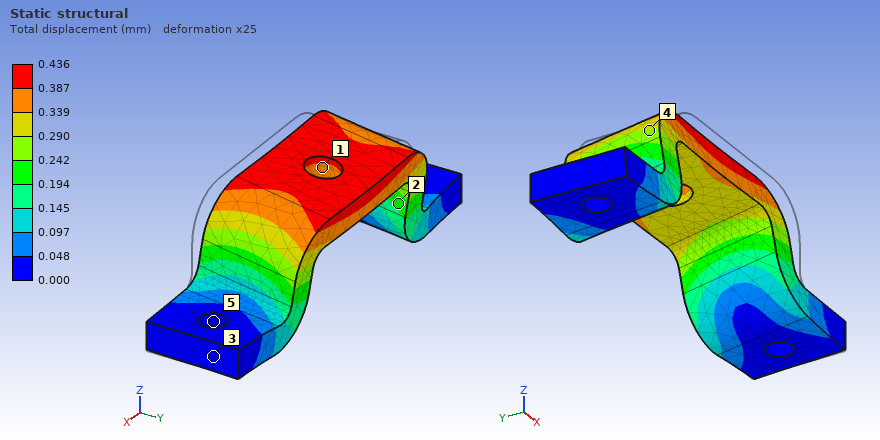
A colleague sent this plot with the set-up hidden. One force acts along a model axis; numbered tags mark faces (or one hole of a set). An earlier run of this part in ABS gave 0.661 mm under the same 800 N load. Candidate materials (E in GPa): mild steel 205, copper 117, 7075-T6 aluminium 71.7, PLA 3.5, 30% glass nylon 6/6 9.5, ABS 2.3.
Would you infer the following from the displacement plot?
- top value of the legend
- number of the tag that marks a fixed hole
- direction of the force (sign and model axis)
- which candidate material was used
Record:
0.436 mm
5
+Y
PLA
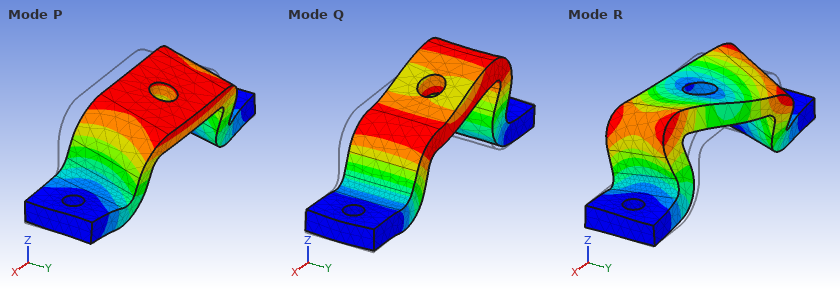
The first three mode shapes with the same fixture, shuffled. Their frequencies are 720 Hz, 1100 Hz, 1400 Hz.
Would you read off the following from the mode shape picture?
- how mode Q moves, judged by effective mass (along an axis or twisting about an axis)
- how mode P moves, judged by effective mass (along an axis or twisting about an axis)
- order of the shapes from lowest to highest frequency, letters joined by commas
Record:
along X
along Y
P, Q, R
